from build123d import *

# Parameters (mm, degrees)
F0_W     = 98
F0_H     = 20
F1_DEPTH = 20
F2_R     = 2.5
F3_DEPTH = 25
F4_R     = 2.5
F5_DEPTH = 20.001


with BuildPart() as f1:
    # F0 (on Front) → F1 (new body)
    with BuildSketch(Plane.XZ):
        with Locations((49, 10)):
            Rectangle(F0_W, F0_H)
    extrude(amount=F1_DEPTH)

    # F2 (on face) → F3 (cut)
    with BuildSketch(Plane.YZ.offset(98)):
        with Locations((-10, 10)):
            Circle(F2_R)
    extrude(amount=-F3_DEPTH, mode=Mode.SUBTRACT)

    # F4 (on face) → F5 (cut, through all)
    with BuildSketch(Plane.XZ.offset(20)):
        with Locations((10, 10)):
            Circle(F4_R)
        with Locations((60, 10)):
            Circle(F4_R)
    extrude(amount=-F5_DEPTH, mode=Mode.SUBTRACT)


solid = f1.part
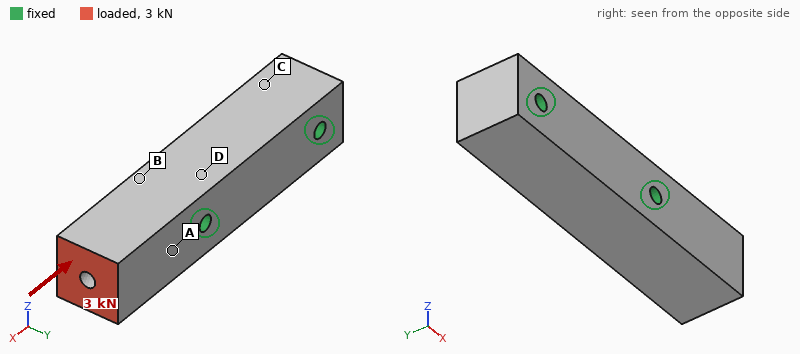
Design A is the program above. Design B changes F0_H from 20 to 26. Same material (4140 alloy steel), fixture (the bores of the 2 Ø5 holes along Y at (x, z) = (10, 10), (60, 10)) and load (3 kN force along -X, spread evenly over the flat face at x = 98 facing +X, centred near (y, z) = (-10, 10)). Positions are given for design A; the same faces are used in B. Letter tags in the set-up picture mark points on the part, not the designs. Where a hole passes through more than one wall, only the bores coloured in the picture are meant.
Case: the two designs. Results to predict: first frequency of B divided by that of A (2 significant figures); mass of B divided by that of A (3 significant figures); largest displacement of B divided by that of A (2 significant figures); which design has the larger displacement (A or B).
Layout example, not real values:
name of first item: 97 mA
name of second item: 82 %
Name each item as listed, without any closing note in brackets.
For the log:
first frequency of B divided by that of A: 1.1
mass of B divided by that of A: 1.31
largest displacement of B divided by that of A: 0.81
which design has the larger displacement: A
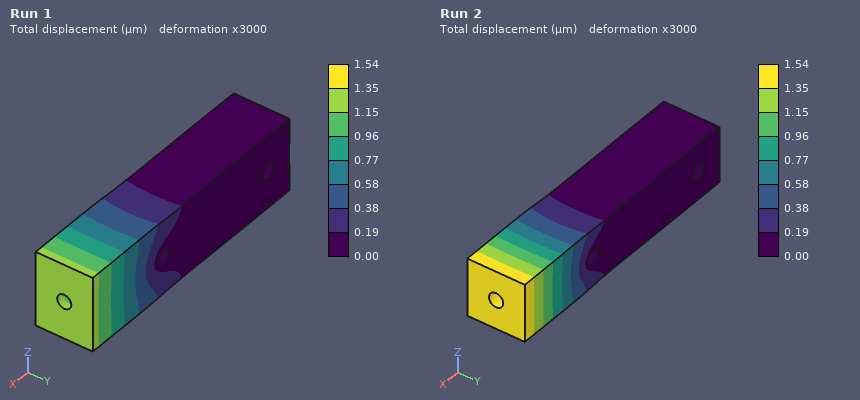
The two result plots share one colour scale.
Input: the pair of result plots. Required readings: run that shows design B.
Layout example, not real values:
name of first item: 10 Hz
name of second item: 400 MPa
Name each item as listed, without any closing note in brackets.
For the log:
run that shows design B: Run 1
